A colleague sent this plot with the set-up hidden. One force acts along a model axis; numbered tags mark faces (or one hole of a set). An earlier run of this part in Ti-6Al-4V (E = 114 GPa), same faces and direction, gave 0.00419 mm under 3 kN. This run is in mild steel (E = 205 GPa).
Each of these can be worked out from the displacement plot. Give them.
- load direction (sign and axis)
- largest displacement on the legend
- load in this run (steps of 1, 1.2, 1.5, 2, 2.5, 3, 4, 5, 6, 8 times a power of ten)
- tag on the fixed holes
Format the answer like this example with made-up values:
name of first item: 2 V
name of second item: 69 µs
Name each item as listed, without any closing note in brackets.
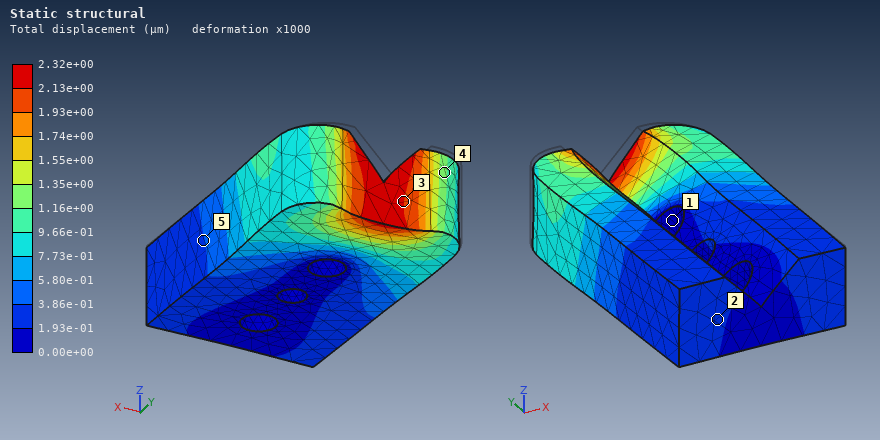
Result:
load direction: -Y
largest displacement on the legend: 2.32e+00 µm
load in this run: 3 kN
tag on the fixed holes: 1
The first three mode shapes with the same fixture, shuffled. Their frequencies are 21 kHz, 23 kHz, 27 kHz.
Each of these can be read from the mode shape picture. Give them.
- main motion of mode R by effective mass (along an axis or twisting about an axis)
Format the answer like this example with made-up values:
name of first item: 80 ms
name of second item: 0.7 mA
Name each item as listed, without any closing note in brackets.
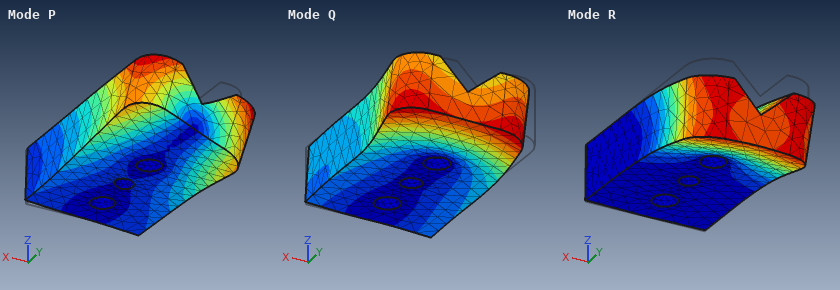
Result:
main motion of mode R by effective mass: along Z
